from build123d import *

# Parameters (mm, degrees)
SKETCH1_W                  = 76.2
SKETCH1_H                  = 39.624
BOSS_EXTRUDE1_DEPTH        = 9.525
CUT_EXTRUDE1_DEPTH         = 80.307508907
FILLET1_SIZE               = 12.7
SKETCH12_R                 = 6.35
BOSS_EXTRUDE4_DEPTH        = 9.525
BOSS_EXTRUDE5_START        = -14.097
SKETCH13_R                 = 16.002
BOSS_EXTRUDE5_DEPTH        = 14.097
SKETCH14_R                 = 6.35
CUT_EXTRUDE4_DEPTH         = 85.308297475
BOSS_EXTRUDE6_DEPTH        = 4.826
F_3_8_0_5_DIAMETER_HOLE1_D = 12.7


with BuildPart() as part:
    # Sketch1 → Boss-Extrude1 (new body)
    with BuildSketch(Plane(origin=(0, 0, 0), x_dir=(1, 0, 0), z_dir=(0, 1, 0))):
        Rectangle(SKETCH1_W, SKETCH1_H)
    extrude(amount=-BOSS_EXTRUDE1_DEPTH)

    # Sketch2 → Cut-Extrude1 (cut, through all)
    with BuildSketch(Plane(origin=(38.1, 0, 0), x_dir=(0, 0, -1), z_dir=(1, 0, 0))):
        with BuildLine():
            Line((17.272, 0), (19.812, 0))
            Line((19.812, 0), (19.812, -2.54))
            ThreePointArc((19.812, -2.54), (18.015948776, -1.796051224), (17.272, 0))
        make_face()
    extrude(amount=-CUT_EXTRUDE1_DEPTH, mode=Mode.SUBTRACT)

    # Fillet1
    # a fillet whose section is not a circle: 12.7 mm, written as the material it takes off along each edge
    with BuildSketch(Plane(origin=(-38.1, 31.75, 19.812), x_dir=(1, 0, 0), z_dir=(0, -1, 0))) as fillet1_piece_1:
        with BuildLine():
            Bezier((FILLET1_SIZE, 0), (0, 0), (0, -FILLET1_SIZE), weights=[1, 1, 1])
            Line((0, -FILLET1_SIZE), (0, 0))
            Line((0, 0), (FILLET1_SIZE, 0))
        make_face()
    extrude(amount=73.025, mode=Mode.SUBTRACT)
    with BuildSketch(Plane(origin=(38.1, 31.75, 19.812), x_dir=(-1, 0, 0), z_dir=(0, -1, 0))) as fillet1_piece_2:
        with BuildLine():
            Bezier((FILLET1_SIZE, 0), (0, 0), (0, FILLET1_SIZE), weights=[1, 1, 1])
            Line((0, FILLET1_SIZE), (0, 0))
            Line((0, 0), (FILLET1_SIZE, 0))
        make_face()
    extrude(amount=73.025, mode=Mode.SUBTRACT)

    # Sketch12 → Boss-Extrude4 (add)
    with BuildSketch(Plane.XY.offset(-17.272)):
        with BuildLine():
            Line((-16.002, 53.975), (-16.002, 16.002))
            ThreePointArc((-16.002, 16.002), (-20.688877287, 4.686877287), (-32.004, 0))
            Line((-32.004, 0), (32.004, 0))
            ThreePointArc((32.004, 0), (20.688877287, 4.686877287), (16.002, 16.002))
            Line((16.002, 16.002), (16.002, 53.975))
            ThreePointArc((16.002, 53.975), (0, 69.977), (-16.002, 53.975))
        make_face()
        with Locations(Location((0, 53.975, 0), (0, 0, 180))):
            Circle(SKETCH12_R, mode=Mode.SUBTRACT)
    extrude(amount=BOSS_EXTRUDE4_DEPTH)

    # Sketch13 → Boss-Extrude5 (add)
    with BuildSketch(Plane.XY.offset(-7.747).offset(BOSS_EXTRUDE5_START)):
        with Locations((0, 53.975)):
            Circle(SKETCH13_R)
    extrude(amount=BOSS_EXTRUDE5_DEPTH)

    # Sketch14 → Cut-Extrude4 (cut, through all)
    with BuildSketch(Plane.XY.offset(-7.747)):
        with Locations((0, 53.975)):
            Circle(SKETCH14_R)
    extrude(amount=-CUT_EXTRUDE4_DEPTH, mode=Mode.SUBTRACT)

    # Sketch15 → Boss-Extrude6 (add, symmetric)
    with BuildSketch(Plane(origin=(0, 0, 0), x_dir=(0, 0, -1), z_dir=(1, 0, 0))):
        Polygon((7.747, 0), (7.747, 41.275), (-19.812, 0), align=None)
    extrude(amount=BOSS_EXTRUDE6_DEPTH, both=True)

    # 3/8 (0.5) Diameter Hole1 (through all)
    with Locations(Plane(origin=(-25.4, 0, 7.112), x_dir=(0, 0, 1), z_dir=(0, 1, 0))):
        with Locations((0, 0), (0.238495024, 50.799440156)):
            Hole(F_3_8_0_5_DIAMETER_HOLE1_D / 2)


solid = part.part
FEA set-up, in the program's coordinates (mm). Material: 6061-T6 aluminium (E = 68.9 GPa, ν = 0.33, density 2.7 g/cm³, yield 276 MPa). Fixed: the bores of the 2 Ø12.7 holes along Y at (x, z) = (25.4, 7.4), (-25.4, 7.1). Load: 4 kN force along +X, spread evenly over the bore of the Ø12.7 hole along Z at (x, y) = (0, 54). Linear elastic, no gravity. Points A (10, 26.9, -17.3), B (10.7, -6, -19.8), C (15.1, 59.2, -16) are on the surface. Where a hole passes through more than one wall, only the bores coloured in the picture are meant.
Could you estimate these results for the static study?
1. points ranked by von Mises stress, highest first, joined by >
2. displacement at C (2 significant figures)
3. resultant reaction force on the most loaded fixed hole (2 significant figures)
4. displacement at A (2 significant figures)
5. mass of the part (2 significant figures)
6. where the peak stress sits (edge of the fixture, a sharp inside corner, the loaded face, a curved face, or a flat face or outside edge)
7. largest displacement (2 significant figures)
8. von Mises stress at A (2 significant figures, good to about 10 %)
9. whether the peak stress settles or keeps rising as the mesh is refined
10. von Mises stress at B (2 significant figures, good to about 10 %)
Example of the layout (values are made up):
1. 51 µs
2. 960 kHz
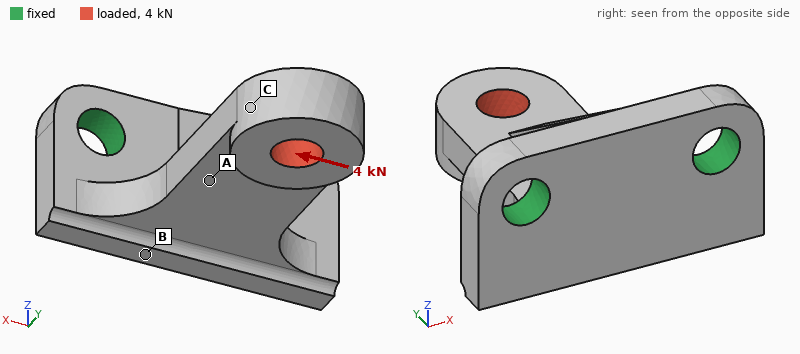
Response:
1. A > B > C
2. 0.26 mm
3. 5.7 kN
4. 0.096 mm
5. 150 g
6. edge of the fixture
7. 0.30 mm
8. 57 MPa
9. keeps rising
10. 37 MPa
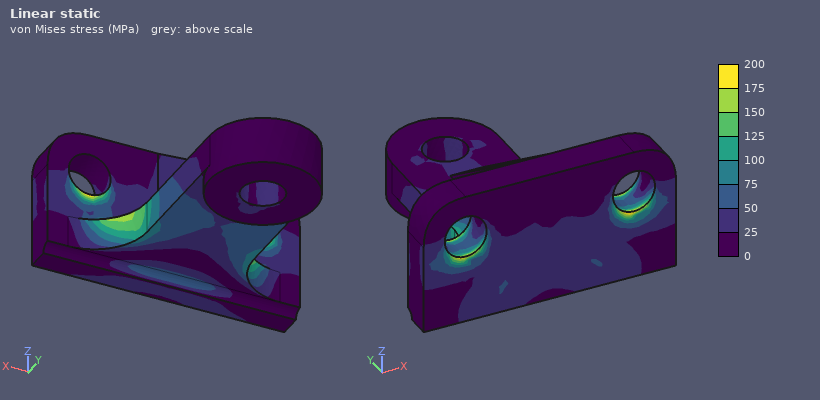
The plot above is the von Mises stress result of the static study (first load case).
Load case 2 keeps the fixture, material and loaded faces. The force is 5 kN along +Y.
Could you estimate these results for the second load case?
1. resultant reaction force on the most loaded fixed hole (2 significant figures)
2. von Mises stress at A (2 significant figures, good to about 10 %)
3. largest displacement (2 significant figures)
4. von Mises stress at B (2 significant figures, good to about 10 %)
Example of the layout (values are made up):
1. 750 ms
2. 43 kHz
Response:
1. 2.6 kN
2. 31 MPa
3. 0.21 mm
4. 11 MPa
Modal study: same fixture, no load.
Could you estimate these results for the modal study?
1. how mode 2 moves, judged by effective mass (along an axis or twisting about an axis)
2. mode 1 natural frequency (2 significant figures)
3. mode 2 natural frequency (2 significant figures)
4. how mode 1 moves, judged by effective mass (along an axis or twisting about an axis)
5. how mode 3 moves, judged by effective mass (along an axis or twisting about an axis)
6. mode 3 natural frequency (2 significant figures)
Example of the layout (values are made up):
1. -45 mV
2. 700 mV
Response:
1. along X
2. 2300 Hz
3. 3700 Hz
4. along Z
5. along Y
6. 7300 Hz
